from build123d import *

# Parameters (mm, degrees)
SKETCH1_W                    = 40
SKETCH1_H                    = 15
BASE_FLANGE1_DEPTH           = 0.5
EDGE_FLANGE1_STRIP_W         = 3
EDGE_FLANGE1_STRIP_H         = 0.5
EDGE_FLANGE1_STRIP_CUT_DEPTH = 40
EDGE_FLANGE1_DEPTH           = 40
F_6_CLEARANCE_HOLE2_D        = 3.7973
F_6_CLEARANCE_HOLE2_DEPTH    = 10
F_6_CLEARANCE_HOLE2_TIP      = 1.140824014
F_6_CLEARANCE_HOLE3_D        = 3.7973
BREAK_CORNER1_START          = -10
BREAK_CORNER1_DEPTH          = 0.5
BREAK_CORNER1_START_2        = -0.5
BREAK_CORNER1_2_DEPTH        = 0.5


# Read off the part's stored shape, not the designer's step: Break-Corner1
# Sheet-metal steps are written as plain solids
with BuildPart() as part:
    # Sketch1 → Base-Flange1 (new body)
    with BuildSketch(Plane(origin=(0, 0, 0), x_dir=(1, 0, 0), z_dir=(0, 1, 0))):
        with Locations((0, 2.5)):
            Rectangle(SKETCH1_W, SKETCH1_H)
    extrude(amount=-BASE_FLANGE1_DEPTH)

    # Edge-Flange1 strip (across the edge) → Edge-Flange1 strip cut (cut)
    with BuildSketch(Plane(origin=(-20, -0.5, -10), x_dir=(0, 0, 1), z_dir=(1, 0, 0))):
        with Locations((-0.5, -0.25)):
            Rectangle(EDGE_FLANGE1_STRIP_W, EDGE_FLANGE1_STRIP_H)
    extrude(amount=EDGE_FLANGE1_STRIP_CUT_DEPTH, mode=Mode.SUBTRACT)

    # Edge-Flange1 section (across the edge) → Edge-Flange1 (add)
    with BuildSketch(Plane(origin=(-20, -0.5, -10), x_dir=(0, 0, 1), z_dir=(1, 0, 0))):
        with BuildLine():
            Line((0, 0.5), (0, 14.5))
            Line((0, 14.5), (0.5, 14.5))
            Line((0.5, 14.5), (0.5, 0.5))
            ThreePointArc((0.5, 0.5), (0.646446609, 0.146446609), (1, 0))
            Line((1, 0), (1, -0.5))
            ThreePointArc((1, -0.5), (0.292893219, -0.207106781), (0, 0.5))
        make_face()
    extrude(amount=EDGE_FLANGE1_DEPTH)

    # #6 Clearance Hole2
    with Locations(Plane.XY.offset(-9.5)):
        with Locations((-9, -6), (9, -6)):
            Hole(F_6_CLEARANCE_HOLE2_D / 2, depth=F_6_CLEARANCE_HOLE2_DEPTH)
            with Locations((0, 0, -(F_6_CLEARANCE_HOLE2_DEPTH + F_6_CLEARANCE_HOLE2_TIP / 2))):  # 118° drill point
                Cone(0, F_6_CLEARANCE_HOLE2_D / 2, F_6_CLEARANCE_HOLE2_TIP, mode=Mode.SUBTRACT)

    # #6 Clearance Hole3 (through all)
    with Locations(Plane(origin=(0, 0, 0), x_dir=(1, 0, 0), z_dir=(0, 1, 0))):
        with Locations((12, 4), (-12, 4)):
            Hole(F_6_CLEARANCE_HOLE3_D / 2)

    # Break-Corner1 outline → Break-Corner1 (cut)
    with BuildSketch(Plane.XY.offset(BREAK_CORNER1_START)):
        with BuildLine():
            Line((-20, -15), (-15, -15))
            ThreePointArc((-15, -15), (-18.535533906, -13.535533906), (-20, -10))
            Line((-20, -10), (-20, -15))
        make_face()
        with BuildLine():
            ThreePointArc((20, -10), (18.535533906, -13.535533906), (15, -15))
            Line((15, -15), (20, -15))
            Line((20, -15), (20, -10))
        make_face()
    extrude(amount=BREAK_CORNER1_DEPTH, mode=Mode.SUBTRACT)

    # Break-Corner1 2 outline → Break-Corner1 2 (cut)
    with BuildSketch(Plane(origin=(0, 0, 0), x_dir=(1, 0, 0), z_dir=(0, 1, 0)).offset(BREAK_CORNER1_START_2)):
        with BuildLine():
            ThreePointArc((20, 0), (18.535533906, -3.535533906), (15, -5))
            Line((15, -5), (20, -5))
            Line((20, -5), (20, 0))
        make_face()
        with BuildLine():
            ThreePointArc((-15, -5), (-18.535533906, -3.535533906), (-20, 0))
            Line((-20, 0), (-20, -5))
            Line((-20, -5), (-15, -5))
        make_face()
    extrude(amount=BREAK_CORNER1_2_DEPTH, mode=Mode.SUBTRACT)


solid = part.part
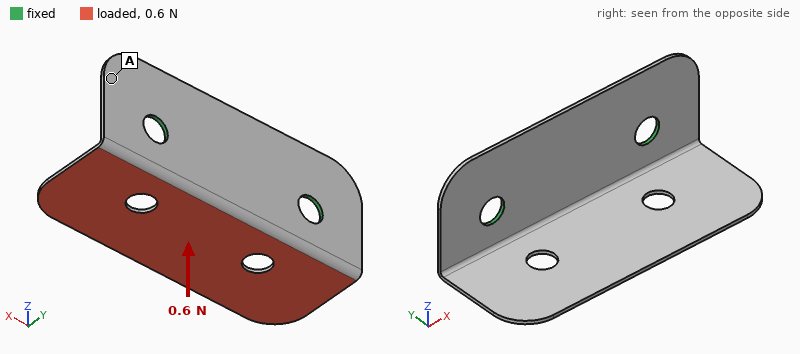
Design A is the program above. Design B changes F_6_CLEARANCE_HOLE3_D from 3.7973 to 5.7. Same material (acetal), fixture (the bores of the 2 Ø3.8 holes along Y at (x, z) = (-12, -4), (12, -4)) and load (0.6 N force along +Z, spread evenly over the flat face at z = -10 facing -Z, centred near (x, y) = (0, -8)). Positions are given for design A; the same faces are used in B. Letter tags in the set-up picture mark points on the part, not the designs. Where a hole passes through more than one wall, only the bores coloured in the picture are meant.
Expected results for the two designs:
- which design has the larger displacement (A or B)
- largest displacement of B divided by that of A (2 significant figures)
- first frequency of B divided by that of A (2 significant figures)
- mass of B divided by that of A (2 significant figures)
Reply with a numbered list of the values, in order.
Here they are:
1. A
2. 0.86
3. 1.1
4. 0.97
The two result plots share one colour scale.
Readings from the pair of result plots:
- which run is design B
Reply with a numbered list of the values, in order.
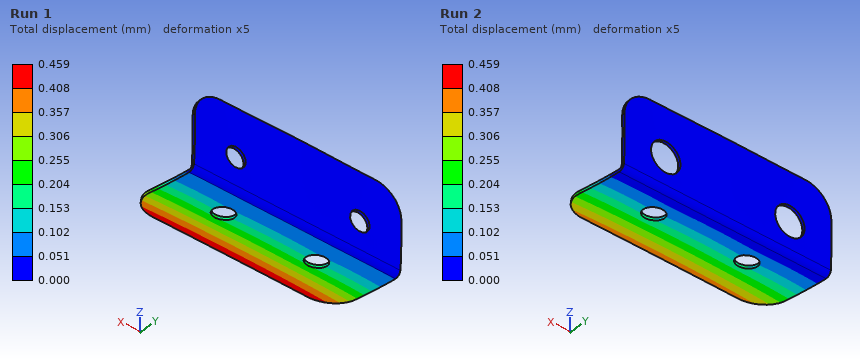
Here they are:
1. Run 2
